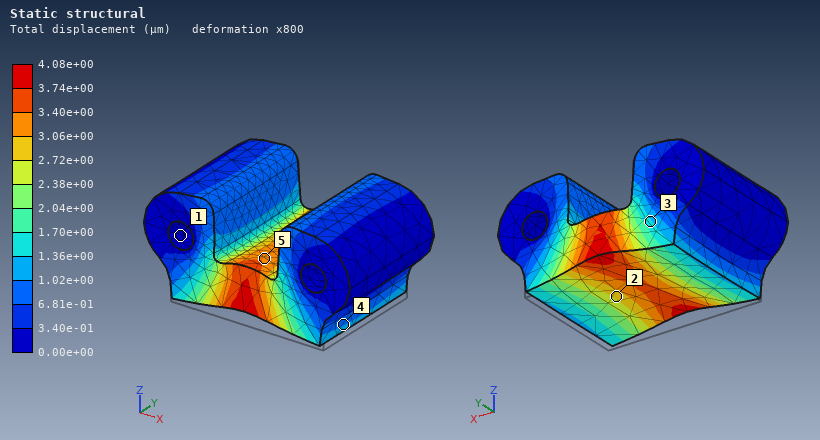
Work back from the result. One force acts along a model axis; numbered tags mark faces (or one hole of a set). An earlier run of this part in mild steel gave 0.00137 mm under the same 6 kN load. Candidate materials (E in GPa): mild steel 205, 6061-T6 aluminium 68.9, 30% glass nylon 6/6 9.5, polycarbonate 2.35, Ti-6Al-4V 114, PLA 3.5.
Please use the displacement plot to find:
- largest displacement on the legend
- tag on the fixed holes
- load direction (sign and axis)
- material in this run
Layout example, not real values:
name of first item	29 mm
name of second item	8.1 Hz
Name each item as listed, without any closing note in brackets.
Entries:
largest displacement on the legend	4.08e+00 µm
tag on the fixed holes	1
load direction	+Z
material in this run	6061-T6 aluminium
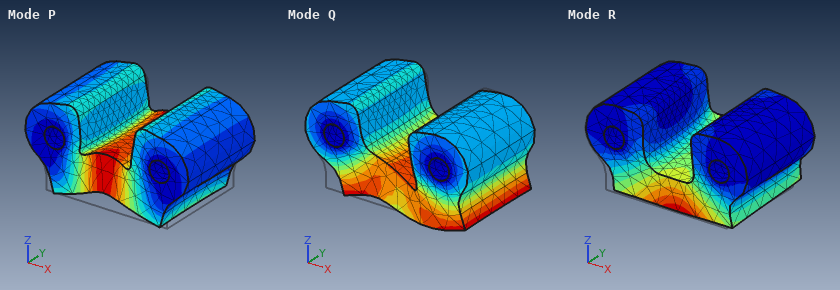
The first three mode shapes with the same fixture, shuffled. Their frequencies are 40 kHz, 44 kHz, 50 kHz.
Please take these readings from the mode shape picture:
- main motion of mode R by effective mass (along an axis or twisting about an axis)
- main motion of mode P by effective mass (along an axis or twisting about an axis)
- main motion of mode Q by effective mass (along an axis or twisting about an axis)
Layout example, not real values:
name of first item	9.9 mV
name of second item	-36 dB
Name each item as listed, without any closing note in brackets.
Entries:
main motion of mode R by effective mass	along Y
main motion of mode P by effective mass	along Z
main motion of mode Q by effective mass	along X
